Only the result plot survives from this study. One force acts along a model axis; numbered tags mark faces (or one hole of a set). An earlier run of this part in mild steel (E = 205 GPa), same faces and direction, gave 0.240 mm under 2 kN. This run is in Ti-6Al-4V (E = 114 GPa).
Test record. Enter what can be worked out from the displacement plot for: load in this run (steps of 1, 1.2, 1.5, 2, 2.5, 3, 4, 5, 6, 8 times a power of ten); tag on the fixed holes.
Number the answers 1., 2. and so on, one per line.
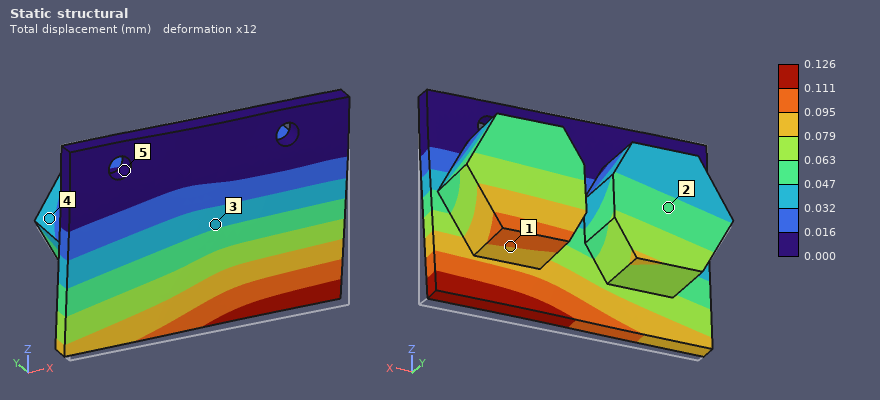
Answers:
1. 600 N
2. 5
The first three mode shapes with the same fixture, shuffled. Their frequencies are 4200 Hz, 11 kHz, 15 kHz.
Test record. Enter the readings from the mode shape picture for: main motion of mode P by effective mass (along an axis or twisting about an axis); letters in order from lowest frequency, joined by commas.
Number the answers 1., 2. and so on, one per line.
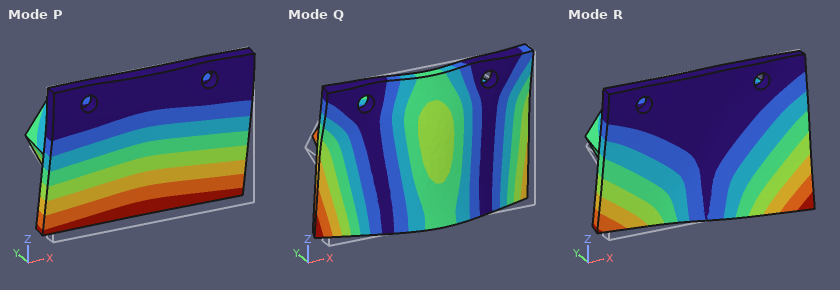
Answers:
1. along Y
2. P, R, Q
